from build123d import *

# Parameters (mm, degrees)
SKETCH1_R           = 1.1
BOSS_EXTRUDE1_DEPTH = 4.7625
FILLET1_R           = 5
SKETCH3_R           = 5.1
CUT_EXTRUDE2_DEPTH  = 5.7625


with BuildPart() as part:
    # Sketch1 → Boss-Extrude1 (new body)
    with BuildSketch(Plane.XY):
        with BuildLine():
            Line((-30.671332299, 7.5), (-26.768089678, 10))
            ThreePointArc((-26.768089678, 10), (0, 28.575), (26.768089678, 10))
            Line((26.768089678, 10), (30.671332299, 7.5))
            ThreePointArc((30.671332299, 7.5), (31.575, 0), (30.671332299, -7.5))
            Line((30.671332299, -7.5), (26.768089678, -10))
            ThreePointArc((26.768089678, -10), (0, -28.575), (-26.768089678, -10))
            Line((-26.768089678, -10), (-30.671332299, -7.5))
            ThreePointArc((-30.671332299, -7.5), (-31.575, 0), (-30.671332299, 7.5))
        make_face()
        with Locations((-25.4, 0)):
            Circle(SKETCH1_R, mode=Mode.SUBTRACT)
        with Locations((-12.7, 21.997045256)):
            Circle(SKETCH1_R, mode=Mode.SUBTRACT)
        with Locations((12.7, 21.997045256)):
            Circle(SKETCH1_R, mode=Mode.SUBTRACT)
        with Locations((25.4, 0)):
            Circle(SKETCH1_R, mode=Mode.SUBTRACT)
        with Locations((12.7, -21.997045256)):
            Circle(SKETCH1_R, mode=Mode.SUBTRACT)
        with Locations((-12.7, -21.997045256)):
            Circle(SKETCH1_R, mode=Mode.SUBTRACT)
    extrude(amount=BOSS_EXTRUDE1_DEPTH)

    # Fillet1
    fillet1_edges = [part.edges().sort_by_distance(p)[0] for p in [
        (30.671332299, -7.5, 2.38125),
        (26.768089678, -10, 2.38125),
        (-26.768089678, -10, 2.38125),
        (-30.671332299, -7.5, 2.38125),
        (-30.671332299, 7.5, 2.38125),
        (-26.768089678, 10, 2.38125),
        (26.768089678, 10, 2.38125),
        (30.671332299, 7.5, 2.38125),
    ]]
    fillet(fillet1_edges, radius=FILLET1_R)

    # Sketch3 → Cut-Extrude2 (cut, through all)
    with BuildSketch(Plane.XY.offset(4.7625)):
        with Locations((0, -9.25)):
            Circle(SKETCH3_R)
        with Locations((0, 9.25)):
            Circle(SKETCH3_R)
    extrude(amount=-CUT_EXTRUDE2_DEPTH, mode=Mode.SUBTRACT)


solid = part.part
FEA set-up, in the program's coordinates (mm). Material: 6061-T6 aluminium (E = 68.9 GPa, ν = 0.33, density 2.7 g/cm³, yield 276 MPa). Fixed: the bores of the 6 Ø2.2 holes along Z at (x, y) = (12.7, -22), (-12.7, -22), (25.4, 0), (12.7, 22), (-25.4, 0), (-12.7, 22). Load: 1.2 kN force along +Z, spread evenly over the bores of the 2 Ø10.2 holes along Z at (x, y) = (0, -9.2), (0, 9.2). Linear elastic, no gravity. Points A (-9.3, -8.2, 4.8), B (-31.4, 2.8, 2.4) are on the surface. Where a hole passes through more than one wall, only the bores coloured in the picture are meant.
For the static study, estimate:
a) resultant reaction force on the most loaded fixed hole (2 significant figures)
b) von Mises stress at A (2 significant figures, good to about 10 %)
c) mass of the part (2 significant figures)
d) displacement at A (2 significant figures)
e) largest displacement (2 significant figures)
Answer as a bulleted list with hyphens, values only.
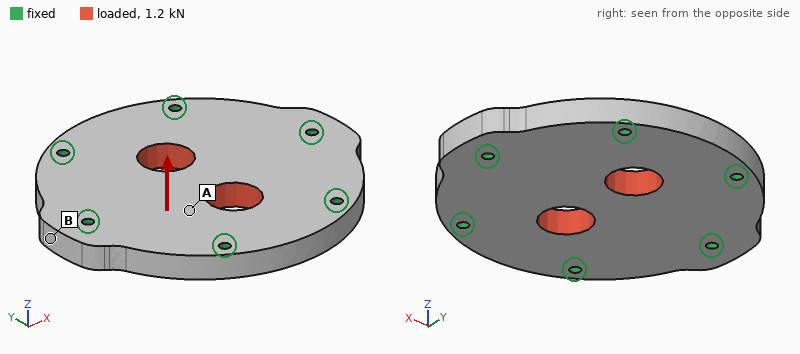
- 240 N
- 19 MPa
- 32 g
- 17 µm
- 30 µm
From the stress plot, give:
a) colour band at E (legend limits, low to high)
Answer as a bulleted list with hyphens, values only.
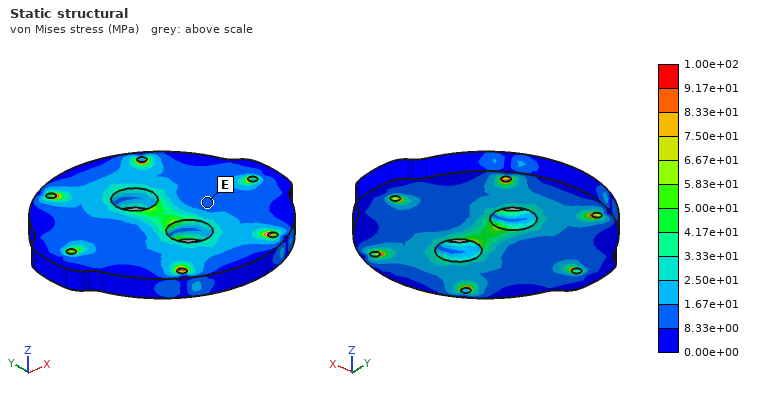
- 8.33e+00 to 1.67e+01 MPa
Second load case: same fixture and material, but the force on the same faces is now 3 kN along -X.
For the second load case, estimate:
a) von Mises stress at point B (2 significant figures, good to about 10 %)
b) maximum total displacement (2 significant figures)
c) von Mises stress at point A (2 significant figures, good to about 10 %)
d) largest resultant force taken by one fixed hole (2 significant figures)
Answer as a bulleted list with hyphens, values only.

- 5.4 MPa
- 3.8 µm
- 8.0 MPa
- 670 N
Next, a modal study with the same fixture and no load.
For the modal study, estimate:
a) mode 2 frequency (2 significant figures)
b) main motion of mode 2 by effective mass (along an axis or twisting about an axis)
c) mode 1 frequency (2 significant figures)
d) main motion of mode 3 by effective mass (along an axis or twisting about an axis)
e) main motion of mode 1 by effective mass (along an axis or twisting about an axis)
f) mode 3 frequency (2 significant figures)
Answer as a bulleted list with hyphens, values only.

- 24 kHz
- twisting about Y
- 13 kHz
- twisting about X
- along Z
- 25 kHz
